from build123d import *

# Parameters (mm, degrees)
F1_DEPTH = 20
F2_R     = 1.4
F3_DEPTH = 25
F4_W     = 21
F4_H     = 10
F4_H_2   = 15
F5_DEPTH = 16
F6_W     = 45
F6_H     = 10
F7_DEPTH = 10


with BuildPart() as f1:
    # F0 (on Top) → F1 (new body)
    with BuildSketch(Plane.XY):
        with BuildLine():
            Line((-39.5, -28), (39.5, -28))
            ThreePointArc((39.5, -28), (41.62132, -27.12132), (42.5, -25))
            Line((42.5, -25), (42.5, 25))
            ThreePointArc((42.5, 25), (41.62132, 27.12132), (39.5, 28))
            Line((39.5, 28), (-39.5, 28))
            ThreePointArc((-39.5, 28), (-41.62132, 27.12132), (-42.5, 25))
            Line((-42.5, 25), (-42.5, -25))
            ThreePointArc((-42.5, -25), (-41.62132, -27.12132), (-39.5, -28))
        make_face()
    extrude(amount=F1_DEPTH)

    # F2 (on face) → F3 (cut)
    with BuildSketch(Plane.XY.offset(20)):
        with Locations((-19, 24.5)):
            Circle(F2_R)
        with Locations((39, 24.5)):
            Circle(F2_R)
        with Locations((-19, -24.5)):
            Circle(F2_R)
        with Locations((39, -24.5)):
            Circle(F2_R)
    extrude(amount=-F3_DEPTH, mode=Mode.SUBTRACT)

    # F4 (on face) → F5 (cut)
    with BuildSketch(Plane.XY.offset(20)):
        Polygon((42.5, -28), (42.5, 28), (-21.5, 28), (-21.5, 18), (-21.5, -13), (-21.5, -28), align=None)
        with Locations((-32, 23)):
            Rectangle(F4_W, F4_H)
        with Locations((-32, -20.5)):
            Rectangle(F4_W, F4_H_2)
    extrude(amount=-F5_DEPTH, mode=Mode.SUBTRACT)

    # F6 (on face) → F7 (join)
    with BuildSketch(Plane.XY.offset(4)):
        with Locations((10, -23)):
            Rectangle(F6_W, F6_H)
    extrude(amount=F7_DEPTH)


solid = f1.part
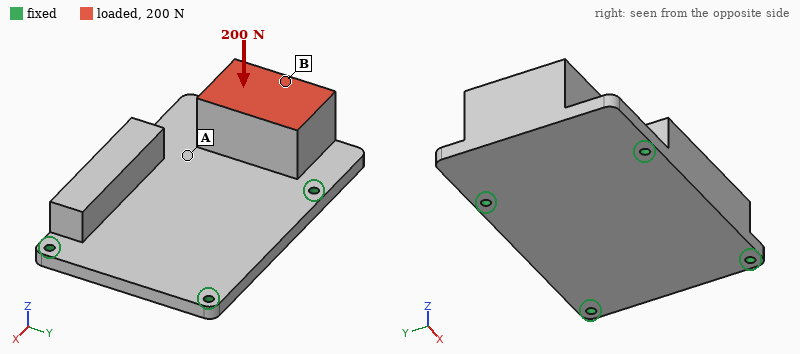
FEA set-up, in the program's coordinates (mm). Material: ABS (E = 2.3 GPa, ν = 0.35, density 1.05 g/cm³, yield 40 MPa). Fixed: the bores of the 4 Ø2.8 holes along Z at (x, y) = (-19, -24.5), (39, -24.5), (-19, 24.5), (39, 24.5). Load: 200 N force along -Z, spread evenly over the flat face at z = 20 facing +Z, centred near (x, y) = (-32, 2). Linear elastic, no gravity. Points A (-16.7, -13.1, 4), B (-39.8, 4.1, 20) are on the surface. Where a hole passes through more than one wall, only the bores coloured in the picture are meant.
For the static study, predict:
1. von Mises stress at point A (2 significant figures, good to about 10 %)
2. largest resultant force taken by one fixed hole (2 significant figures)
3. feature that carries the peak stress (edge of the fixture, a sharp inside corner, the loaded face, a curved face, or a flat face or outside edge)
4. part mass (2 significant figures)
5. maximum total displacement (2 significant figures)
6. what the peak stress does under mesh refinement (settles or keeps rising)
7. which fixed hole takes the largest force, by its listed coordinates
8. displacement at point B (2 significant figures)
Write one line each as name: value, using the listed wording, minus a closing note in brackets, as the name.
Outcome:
von Mises stress at point A: 8.9 MPa
largest resultant force taken by one fixed hole: 120 N
feature that carries the peak stress: edge of the fixture
part mass: 36 g
maximum total displacement: 0.97 mm
what the peak stress does under mesh refinement: keeps rising
which fixed hole takes the largest force, by its listed coordinates: (-19, 24.5)
displacement at point B: 0.88 mm
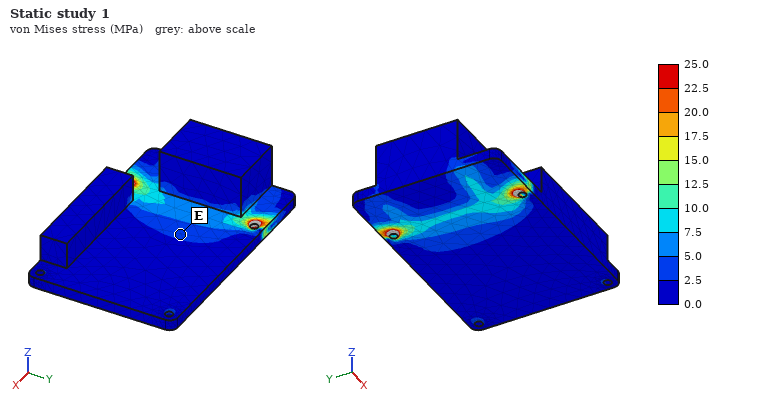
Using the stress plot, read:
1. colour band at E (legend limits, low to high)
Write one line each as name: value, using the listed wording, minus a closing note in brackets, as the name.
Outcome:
colour band at E: 2.5 to 5.0 MPa
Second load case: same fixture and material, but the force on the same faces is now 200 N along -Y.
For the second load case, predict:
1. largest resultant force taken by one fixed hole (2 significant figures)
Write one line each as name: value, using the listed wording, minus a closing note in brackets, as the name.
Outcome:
largest resultant force taken by one fixed hole: 140 N
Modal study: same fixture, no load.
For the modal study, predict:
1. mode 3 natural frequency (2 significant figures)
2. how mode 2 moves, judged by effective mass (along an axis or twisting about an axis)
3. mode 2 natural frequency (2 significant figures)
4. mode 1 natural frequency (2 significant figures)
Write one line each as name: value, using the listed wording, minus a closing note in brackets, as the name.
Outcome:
mode 3 natural frequency: 2100 Hz
how mode 2 moves, judged by effective mass: along Z
mode 2 natural frequency: 1400 Hz
mode 1 natural frequency: 660 Hz
